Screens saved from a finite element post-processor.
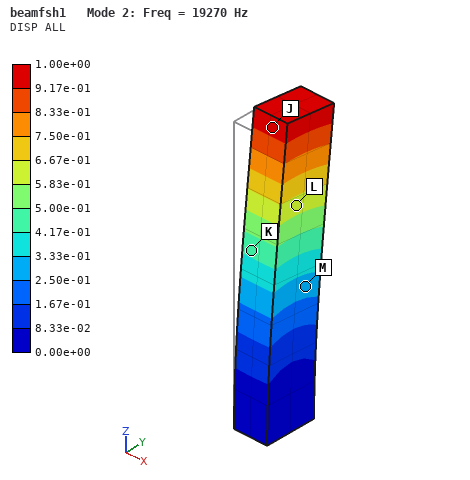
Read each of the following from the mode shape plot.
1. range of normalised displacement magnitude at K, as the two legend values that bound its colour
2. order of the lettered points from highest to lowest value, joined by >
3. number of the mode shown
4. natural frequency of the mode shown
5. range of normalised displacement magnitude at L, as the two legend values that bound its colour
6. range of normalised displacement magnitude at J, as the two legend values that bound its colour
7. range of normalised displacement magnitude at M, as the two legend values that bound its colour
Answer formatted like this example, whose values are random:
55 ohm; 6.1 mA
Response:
4.17e-01 to 5.00e-01; J > L > K > M; 2; 19270 Hz; 5.83e-01 to 6.67e-01; 9.17e-01 to 1.00e+00; 2.50e-01 to 3.33e-01
